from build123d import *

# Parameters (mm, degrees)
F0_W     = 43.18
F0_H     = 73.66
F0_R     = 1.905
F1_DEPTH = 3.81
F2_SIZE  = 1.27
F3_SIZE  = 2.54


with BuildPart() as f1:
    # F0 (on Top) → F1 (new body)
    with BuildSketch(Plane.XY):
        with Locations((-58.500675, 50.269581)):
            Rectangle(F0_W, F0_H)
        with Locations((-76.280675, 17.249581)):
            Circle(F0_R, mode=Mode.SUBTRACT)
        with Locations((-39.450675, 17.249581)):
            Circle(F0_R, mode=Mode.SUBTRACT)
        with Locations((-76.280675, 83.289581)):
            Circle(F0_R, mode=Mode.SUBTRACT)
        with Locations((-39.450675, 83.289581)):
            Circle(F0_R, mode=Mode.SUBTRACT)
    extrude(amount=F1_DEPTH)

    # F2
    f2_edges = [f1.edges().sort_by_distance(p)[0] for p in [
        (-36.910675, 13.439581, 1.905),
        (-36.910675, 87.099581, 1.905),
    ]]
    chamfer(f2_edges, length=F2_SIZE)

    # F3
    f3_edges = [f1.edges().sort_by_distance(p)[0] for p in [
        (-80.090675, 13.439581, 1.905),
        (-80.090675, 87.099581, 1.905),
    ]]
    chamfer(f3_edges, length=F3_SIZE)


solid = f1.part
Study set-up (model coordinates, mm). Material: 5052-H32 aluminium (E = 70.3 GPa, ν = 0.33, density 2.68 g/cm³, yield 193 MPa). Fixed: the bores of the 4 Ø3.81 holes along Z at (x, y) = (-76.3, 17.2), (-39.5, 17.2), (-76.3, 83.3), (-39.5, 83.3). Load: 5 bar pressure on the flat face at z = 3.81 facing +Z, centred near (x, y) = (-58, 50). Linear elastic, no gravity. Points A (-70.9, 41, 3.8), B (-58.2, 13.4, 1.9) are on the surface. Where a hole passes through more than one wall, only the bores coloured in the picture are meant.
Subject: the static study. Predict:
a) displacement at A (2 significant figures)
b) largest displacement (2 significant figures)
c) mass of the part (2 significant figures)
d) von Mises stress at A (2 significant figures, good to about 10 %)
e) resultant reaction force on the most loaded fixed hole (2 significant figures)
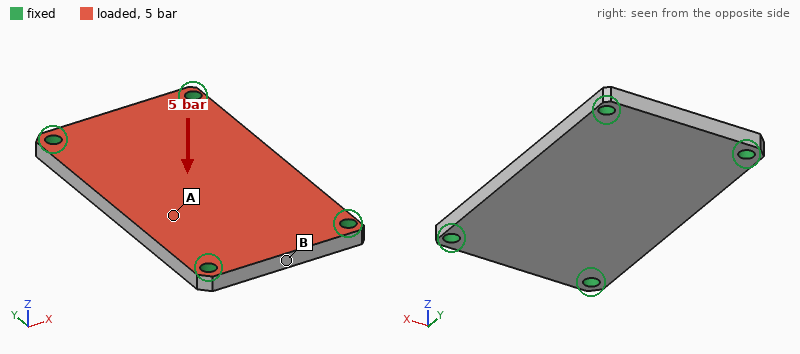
0.087 mm
0.10 mm
32 g
33 MPa
400 N
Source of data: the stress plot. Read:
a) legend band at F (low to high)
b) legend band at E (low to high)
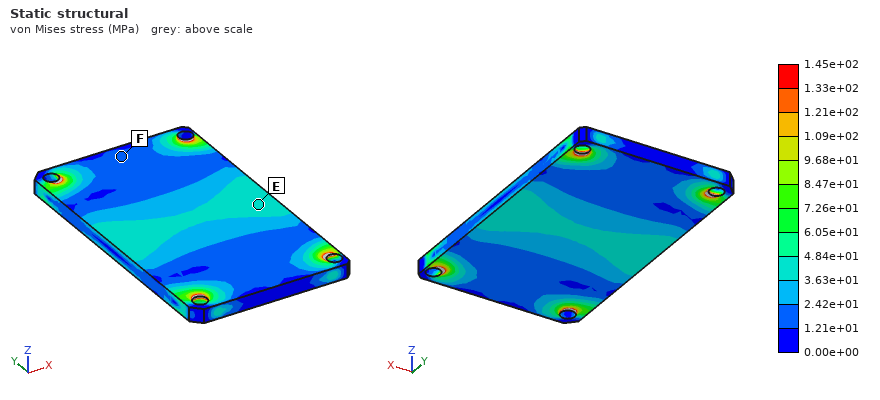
1.21e+01 to 2.42e+01 MPa
3.63e+01 to 4.84e+01 MPa
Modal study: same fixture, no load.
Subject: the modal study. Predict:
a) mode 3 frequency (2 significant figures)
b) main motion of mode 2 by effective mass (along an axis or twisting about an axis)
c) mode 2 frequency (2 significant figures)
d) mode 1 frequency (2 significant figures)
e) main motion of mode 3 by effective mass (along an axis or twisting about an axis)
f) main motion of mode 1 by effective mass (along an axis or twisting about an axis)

10 kHz
twisting about Y
6500 Hz
4000 Hz
twisting about X
along Z
